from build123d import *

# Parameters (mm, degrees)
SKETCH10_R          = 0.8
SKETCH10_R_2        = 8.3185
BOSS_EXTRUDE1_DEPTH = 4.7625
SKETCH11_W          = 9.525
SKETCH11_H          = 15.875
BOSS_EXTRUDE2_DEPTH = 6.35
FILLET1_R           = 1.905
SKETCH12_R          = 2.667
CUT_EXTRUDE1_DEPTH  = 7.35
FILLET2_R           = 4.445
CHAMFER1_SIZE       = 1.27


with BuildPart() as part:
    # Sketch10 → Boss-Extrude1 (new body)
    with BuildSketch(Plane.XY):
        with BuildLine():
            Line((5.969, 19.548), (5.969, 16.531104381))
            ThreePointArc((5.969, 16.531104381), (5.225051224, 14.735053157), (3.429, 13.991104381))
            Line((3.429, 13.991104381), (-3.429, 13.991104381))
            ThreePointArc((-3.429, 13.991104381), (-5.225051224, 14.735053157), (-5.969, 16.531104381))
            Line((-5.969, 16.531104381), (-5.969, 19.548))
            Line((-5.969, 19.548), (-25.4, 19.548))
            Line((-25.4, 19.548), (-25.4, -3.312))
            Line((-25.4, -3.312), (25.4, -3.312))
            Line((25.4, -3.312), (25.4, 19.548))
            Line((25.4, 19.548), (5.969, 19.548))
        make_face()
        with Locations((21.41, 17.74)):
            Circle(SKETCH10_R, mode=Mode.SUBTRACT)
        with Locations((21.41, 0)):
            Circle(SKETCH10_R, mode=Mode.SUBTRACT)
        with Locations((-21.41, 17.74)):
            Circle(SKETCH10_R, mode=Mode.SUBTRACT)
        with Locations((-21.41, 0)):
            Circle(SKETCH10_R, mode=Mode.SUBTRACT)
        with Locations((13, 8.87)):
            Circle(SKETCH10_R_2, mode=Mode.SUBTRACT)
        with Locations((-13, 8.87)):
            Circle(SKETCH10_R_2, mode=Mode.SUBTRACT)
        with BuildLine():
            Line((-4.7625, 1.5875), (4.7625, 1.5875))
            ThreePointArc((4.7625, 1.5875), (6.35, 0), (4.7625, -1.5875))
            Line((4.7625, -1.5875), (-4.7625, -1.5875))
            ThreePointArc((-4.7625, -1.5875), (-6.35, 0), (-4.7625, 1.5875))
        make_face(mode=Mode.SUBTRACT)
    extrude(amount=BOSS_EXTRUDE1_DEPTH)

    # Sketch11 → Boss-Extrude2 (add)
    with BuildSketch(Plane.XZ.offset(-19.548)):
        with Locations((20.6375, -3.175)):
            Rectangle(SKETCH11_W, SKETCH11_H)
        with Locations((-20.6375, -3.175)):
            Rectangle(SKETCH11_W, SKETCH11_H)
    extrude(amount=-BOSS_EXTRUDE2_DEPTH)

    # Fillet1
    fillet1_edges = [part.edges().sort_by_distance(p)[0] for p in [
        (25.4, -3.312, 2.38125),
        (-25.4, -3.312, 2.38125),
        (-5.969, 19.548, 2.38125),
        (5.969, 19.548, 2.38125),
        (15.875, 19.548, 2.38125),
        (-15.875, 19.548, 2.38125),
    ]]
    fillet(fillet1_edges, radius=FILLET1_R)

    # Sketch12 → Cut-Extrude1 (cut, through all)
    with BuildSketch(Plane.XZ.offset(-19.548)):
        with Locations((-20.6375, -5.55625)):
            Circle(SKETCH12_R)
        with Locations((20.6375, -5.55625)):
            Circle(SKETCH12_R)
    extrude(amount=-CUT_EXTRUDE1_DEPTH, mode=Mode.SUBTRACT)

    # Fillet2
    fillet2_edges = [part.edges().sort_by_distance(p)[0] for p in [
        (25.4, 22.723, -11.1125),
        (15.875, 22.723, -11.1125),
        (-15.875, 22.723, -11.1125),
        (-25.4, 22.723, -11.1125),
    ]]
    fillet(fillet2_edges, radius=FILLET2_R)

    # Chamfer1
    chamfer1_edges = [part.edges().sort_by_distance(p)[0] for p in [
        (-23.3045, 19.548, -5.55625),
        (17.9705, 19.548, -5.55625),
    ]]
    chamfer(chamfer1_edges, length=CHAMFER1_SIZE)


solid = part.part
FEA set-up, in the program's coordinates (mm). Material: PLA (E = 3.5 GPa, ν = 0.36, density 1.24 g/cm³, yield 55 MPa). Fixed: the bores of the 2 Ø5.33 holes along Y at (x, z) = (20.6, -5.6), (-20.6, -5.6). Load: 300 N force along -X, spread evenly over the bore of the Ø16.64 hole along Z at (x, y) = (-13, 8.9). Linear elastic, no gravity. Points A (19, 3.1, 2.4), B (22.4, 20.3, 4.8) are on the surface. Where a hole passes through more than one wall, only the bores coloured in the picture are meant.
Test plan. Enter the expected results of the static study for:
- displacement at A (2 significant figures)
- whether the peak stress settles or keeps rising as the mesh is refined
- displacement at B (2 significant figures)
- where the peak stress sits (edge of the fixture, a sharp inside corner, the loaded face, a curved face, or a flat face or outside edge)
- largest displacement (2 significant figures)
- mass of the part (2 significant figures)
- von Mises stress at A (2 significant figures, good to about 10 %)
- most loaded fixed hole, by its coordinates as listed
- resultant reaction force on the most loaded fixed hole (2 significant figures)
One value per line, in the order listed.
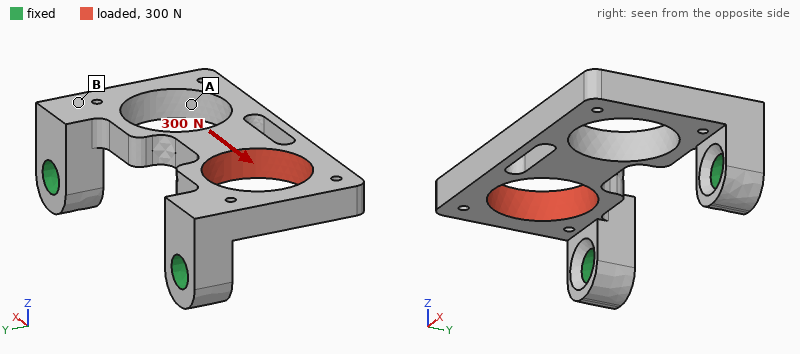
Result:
0.17 mm
keeps rising
0.040 mm
edge of the fixture
0.24 mm
5.5 g
10.0 MPa
(-20.6, -5.6)
220 N
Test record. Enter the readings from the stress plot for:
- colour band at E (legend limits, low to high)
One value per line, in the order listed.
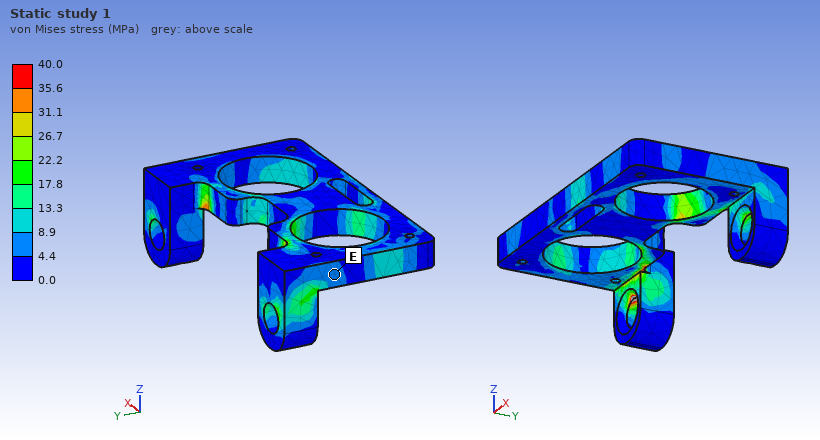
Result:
4.4 to 8.9 MPa
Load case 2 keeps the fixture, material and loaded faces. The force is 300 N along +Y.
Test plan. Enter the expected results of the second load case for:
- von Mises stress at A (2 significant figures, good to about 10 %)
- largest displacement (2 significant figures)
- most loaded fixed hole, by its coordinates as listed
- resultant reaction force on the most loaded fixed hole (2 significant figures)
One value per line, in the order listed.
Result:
4.2 MPa
0.34 mm
(-20.6, -5.6)
250 N
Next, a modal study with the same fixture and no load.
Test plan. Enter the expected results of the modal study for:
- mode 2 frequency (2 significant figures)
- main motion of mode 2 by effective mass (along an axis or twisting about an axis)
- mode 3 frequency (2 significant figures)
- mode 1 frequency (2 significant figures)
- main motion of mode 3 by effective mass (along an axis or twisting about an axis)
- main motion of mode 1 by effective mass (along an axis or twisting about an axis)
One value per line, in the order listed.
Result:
2100 Hz
twisting about Y
3200 Hz
1000 Hz
along X
along Z
